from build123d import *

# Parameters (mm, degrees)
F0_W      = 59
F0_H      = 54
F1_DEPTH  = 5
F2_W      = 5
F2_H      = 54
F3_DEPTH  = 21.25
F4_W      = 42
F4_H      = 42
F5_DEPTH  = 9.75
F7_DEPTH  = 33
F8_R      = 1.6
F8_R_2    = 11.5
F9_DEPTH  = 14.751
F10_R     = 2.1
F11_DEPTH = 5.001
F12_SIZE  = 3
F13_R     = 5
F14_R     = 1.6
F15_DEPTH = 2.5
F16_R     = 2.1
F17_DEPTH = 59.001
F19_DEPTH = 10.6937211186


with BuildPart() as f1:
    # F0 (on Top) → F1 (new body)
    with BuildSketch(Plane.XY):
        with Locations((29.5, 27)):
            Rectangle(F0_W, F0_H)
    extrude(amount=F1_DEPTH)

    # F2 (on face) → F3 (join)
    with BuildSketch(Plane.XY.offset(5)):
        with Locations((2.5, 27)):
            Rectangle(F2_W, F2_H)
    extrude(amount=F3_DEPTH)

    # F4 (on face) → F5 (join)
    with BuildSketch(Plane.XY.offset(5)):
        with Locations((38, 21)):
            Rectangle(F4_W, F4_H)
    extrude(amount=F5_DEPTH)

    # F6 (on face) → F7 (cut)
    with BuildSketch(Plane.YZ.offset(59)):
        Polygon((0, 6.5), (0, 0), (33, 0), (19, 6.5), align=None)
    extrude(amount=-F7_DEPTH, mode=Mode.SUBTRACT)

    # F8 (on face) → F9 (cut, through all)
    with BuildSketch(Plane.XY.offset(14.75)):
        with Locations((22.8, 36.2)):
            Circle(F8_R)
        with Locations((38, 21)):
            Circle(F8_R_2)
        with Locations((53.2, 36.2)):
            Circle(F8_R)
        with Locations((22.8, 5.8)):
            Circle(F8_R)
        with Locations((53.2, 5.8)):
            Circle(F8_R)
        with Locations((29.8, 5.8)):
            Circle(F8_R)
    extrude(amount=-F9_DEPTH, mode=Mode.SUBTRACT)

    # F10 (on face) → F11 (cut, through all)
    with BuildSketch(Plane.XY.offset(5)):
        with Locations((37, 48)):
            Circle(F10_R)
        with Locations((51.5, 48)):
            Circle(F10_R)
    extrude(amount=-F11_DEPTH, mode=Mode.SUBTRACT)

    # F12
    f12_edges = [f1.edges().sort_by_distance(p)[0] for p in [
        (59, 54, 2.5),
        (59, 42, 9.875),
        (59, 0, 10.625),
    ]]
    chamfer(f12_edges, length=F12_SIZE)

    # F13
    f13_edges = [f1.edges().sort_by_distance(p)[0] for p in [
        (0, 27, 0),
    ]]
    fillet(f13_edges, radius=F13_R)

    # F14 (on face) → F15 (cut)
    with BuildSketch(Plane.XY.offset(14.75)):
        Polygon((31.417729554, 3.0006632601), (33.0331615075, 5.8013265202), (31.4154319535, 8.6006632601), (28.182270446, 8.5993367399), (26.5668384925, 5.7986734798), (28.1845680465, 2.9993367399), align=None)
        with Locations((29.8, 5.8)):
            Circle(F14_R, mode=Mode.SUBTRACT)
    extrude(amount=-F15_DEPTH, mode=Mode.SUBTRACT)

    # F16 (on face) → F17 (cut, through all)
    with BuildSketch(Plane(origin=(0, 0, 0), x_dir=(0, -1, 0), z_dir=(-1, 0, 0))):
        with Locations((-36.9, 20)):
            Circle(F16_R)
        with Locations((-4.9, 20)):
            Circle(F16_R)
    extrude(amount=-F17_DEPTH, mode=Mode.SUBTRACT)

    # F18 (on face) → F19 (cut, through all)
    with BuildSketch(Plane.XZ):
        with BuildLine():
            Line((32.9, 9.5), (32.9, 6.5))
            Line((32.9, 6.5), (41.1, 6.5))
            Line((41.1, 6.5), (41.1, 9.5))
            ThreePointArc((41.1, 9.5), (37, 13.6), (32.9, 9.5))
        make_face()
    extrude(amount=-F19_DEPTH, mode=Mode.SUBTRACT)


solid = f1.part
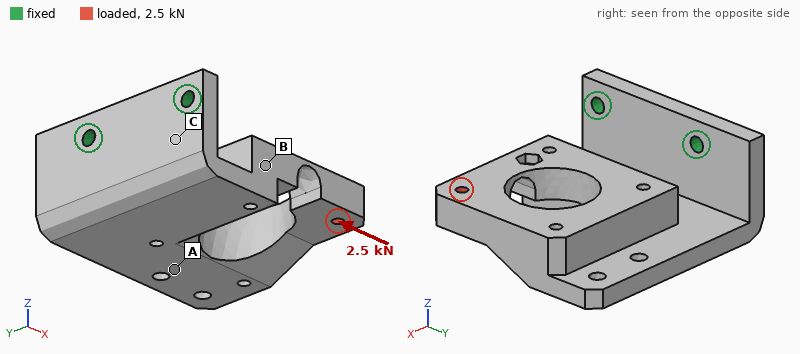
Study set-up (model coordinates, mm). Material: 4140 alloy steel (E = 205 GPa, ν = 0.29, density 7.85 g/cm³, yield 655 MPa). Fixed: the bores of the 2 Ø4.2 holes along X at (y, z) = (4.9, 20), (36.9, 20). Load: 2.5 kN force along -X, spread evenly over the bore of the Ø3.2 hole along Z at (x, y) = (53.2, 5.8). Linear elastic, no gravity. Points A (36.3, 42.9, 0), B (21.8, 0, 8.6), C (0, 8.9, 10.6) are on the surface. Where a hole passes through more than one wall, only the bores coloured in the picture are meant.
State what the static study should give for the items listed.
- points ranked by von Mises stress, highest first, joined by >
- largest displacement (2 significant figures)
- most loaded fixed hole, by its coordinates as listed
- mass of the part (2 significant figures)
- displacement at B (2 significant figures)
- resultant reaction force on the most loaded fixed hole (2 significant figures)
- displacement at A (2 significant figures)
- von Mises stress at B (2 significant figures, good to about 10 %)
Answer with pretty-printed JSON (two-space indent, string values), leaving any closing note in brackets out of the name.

{
  "points ranked by von Mises stress, highest first, joined by >": "C > B > A",
  "largest displacement": "0.16 mm",
  "most loaded fixed hole, by its coordinates as listed": "(4.9, 20)",
  "mass of the part": "220 g",
  "displacement at B": "0.082 mm",
  "resultant reaction force on the most loaded fixed hole": "2.3 kN",
  "displacement at A": "0.072 mm",
  "von Mises stress at B": "51 MPa"
}
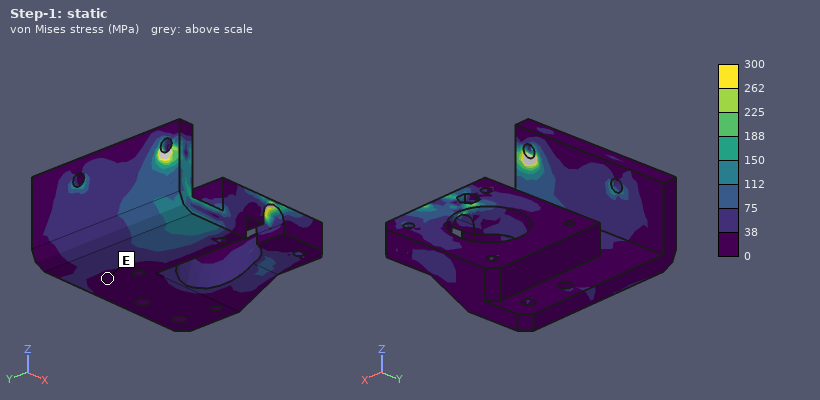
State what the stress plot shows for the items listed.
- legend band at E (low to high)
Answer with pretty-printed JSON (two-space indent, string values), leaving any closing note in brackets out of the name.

{
  "legend band at E": "0 to 38 MPa"
}
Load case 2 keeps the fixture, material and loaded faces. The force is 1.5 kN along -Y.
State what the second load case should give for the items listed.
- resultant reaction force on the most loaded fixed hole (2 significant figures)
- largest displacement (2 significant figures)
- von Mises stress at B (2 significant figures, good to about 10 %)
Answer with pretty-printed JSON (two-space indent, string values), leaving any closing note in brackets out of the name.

{
  "resultant reaction force on the most loaded fixed hole": "2.3 kN",
  "largest displacement": "0.20 mm",
  "von Mises stress at B": "32 MPa"
}
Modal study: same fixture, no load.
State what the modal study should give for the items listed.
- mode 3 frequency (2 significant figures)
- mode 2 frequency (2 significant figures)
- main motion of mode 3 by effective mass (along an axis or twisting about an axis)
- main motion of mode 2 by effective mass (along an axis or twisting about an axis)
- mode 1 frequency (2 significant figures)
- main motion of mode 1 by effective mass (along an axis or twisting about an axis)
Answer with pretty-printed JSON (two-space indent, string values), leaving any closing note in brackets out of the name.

{
  "mode 3 frequency": "3300 Hz",
  "mode 2 frequency": "1700 Hz",
  "main motion of mode 3 by effective mass": "along X",
  "main motion of mode 2 by effective mass": "along Y",
  "mode 1 frequency": "730 Hz",
  "main motion of mode 1 by effective mass": "along Z"
}
